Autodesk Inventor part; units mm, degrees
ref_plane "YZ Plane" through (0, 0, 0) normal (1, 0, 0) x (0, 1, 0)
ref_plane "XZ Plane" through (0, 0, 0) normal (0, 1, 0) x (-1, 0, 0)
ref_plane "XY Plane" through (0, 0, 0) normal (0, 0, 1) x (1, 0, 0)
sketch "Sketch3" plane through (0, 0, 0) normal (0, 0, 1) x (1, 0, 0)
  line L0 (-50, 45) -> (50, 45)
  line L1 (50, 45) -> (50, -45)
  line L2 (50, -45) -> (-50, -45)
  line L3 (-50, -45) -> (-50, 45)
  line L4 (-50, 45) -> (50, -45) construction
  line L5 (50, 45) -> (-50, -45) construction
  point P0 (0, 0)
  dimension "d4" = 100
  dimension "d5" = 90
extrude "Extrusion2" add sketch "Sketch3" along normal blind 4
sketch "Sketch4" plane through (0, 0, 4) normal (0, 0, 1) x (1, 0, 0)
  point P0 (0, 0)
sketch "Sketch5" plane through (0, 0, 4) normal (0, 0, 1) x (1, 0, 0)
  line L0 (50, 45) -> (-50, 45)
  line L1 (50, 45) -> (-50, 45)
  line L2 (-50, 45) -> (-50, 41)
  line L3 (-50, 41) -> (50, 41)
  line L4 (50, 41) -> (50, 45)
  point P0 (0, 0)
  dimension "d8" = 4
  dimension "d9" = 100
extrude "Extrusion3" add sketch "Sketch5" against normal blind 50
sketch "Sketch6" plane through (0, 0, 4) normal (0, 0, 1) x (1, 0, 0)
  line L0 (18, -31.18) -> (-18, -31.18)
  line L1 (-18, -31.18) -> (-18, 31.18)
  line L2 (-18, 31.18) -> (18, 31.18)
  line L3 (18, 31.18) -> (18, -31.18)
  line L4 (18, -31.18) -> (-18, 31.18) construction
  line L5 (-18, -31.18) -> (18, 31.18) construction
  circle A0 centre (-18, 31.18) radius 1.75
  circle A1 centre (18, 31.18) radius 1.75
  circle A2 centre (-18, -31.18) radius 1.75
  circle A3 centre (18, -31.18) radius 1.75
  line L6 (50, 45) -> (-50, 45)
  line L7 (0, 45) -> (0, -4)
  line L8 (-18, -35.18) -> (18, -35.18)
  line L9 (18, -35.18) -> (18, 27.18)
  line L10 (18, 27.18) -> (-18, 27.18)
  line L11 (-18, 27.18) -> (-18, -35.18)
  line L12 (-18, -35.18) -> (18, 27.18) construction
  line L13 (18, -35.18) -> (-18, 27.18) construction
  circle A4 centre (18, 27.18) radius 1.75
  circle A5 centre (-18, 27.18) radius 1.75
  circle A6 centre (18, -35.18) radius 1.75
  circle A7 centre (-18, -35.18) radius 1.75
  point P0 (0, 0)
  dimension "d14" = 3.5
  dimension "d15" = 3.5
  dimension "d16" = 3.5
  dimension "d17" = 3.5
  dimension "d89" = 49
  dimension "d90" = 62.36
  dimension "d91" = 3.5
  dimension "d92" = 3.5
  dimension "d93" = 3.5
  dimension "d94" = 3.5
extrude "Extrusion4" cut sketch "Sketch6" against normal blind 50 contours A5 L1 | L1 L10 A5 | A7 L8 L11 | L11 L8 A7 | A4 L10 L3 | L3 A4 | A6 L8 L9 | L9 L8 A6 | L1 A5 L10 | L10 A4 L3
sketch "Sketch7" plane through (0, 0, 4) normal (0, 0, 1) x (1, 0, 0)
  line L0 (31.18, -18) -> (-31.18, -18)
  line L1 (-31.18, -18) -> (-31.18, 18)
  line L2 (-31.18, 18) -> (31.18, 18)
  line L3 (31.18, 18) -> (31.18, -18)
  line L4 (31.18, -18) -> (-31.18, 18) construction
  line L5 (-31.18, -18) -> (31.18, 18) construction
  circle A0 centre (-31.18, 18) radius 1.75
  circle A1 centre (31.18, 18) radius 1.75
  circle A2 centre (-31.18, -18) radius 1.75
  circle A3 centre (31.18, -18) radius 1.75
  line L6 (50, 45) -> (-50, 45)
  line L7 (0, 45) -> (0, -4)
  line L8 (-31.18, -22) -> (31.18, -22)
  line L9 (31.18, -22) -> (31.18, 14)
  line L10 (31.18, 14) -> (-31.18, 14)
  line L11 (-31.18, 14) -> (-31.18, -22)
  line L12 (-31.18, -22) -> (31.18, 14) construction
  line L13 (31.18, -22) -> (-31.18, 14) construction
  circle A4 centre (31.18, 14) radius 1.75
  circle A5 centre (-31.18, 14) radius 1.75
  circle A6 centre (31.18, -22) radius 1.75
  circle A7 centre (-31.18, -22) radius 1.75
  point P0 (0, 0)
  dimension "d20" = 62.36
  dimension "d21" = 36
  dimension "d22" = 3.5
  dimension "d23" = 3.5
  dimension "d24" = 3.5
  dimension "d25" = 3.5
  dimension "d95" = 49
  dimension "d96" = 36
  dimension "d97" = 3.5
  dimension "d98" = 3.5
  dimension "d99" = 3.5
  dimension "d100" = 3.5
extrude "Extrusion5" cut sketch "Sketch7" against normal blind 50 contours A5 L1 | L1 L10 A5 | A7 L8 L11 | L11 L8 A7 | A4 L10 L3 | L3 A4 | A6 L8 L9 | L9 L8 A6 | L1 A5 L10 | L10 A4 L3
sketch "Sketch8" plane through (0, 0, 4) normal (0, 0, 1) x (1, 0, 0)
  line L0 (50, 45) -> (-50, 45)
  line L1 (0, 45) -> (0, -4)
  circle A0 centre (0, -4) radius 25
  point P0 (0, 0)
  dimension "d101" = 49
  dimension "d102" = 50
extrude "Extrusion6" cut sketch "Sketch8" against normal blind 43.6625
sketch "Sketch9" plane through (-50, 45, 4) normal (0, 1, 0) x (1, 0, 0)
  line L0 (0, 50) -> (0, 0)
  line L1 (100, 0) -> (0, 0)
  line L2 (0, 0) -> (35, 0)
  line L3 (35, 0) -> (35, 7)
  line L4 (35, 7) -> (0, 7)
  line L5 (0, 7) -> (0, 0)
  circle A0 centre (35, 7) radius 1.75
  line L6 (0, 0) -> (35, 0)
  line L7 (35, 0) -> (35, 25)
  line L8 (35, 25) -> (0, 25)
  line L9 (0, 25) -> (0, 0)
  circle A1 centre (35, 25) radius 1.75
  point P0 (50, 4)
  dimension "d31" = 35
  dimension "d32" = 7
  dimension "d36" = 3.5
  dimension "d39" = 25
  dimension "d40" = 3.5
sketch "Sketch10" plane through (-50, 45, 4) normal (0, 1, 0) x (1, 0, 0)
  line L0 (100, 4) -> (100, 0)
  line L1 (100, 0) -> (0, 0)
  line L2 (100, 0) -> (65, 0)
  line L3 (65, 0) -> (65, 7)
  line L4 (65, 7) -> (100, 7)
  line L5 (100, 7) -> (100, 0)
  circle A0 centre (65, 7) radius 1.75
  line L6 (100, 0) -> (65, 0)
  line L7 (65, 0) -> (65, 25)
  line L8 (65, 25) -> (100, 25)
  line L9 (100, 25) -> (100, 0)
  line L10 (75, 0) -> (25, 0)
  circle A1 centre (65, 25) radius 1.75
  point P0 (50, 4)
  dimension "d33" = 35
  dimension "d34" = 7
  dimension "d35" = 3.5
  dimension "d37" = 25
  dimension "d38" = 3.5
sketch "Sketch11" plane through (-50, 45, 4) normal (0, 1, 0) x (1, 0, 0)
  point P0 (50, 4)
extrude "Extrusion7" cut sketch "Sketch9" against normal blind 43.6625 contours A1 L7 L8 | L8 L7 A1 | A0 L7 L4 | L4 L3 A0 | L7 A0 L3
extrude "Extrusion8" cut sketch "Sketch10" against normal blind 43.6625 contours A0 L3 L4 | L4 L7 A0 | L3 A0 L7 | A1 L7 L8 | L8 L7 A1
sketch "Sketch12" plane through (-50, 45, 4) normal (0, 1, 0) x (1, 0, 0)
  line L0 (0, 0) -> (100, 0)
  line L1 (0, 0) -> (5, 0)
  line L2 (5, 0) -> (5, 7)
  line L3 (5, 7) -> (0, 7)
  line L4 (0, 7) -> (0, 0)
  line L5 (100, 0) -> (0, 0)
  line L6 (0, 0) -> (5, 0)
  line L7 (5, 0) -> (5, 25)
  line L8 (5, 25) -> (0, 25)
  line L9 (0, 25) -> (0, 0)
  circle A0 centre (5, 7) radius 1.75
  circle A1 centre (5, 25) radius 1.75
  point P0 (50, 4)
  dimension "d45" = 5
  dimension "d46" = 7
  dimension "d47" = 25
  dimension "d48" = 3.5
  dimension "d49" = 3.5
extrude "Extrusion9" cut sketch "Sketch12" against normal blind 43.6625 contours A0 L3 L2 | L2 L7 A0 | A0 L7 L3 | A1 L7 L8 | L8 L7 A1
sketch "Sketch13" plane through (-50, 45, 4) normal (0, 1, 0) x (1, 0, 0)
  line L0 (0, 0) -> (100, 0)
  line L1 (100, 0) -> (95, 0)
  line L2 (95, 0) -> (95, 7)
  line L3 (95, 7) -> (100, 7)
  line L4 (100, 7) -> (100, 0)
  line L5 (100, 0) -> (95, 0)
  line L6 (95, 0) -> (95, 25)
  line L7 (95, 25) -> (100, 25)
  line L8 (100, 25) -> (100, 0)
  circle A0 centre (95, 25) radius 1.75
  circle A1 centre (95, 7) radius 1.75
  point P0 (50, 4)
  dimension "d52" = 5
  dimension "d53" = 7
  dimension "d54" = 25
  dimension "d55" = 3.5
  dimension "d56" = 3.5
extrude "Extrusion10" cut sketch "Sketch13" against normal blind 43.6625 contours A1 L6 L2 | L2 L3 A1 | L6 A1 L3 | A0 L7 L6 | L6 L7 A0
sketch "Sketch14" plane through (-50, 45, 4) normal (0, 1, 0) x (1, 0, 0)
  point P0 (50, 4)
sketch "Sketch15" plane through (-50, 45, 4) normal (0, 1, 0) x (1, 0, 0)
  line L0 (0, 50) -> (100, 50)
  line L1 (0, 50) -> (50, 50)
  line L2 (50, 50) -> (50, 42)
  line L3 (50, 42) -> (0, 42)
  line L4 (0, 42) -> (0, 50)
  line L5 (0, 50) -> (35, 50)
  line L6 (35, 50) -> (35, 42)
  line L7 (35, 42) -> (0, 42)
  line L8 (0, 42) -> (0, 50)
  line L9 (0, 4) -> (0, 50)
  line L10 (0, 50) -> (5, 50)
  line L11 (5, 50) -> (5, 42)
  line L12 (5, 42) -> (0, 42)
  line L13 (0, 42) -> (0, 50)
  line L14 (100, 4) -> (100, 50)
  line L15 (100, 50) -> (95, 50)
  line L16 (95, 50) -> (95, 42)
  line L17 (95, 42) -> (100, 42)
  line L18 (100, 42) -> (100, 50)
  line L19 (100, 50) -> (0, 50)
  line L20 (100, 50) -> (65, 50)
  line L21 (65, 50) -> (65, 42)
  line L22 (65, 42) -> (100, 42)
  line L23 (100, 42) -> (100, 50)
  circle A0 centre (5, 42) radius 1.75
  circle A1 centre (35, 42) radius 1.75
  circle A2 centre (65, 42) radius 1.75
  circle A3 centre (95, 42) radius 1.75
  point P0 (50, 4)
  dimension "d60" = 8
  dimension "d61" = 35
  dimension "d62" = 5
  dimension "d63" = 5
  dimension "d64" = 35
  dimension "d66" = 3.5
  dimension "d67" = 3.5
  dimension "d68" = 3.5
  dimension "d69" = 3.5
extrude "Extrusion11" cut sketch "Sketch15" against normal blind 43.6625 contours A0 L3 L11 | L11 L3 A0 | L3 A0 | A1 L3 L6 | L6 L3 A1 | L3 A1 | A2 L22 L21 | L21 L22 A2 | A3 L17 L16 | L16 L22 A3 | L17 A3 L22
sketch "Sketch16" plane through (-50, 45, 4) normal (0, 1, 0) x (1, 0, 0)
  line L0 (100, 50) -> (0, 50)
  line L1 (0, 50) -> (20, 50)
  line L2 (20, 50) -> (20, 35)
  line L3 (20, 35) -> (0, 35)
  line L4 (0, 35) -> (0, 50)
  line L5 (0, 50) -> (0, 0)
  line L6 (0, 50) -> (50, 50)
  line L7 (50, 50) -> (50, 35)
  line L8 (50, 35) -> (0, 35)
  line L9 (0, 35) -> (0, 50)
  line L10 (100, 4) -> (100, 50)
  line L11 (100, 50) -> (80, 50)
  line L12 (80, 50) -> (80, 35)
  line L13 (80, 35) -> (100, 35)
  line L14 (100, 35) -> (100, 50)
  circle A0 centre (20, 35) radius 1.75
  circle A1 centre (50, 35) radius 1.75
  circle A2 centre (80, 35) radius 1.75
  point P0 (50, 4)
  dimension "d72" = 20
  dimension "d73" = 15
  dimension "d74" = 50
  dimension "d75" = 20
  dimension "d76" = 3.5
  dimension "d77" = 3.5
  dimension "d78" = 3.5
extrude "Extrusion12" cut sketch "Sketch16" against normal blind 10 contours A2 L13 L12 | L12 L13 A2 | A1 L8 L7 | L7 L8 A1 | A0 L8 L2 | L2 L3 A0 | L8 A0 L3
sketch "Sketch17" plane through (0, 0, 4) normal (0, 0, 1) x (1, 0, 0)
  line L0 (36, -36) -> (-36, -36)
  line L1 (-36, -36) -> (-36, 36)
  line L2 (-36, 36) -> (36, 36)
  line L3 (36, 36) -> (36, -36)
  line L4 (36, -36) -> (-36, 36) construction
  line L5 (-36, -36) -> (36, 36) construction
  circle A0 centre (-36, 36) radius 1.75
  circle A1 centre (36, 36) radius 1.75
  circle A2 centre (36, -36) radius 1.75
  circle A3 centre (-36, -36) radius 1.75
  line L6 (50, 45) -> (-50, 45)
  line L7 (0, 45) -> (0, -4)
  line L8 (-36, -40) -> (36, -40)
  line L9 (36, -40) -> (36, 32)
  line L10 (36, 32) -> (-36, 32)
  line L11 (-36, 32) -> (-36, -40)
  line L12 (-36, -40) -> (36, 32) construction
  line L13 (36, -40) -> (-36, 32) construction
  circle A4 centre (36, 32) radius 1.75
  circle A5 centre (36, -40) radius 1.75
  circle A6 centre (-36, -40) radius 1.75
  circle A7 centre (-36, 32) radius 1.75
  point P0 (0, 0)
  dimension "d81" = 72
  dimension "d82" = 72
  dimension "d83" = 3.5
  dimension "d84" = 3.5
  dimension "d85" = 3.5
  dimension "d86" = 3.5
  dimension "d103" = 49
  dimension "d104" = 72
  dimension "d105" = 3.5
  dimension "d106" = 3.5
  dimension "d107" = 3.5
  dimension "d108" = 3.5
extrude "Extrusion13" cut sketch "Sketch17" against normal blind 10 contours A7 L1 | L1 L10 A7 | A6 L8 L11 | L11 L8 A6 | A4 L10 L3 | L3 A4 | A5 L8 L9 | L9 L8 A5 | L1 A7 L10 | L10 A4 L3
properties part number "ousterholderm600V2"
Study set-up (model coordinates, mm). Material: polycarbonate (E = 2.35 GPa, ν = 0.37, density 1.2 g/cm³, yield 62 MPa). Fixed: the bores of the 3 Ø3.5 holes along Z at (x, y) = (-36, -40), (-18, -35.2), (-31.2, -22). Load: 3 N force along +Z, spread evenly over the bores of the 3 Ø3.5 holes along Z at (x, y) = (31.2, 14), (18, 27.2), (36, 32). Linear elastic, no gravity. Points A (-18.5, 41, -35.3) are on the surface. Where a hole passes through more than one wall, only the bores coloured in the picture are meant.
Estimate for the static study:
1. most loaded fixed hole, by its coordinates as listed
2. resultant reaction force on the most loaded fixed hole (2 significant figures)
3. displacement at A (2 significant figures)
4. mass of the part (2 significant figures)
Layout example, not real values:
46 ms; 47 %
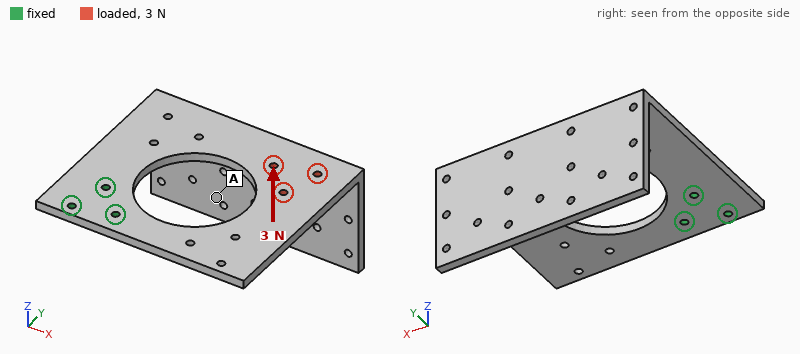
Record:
(-31.2, -22); 3.9 N; 0.78 mm; 55 g
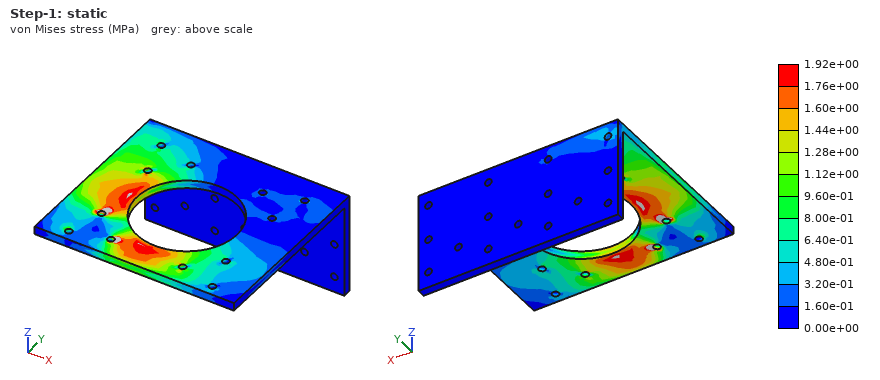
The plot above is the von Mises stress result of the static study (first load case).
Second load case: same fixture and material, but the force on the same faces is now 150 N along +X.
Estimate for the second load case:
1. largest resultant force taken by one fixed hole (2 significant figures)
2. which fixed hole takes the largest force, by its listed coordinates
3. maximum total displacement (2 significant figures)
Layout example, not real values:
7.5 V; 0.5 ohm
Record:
310 N; (-31.2, -22); 0.82 mm
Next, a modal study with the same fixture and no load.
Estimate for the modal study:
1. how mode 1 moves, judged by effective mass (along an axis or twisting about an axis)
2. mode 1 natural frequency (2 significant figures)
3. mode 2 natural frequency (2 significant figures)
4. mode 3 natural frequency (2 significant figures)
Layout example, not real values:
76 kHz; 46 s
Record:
along Z; 47 Hz; 96 Hz; 210 Hz
